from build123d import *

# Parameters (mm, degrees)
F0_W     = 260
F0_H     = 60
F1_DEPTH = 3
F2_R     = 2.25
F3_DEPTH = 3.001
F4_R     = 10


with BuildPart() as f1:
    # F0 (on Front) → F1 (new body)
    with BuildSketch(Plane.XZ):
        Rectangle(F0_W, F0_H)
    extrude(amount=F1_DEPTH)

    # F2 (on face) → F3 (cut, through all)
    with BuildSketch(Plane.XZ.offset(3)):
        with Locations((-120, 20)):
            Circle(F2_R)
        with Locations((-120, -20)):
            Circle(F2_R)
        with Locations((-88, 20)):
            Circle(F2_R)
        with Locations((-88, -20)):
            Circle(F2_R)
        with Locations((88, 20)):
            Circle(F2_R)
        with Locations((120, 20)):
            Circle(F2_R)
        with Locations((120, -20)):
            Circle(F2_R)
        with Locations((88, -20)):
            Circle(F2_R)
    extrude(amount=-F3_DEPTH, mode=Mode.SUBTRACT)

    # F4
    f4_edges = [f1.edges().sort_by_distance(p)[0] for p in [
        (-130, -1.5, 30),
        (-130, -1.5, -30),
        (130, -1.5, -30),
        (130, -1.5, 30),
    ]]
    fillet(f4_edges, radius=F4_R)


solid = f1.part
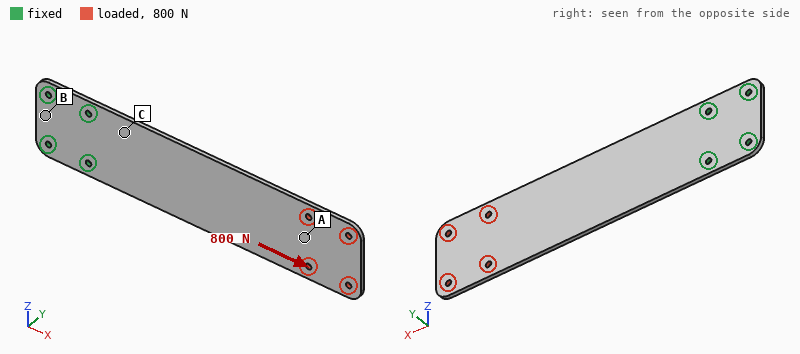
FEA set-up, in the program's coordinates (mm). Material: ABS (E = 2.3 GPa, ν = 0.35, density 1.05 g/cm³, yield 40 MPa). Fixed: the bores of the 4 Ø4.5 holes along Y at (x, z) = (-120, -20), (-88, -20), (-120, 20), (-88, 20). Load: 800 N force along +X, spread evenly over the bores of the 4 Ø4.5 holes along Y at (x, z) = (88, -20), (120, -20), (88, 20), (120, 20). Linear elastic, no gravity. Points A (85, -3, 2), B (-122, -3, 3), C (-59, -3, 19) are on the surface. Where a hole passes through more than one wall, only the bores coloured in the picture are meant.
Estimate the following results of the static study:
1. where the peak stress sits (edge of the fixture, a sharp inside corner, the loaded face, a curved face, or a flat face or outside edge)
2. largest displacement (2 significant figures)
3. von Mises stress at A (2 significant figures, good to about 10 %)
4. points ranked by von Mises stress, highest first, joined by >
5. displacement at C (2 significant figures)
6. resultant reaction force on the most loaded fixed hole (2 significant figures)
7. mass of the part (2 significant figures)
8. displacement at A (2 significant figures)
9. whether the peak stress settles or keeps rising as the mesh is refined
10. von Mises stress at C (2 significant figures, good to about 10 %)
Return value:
edge of the fixture
0.41 mm
3.2 MPa
C > A > B
0.069 mm
330 N
48 g
0.34 mm
keeps rising
4.5 MPa
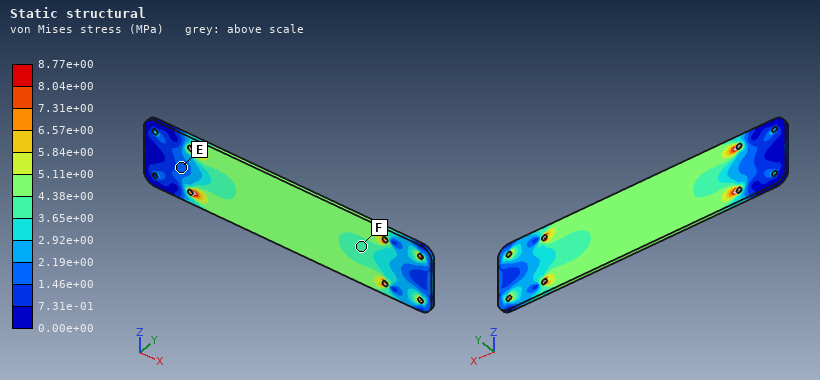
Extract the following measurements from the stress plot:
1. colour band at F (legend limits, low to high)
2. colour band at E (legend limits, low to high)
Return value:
3.65e+00 to 4.38e+00 MPa
1.46e+00 to 2.19e+00 MPa
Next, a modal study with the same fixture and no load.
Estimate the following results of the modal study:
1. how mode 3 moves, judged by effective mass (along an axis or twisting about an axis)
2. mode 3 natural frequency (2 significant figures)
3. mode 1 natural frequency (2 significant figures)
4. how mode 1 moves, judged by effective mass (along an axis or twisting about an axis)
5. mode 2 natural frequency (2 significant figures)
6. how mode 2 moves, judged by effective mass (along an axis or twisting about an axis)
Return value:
twisting about X
110 Hz
15 Hz
along Y
96 Hz
along Y
